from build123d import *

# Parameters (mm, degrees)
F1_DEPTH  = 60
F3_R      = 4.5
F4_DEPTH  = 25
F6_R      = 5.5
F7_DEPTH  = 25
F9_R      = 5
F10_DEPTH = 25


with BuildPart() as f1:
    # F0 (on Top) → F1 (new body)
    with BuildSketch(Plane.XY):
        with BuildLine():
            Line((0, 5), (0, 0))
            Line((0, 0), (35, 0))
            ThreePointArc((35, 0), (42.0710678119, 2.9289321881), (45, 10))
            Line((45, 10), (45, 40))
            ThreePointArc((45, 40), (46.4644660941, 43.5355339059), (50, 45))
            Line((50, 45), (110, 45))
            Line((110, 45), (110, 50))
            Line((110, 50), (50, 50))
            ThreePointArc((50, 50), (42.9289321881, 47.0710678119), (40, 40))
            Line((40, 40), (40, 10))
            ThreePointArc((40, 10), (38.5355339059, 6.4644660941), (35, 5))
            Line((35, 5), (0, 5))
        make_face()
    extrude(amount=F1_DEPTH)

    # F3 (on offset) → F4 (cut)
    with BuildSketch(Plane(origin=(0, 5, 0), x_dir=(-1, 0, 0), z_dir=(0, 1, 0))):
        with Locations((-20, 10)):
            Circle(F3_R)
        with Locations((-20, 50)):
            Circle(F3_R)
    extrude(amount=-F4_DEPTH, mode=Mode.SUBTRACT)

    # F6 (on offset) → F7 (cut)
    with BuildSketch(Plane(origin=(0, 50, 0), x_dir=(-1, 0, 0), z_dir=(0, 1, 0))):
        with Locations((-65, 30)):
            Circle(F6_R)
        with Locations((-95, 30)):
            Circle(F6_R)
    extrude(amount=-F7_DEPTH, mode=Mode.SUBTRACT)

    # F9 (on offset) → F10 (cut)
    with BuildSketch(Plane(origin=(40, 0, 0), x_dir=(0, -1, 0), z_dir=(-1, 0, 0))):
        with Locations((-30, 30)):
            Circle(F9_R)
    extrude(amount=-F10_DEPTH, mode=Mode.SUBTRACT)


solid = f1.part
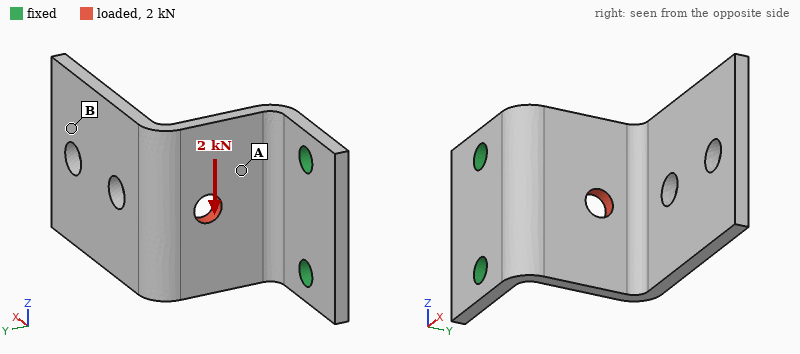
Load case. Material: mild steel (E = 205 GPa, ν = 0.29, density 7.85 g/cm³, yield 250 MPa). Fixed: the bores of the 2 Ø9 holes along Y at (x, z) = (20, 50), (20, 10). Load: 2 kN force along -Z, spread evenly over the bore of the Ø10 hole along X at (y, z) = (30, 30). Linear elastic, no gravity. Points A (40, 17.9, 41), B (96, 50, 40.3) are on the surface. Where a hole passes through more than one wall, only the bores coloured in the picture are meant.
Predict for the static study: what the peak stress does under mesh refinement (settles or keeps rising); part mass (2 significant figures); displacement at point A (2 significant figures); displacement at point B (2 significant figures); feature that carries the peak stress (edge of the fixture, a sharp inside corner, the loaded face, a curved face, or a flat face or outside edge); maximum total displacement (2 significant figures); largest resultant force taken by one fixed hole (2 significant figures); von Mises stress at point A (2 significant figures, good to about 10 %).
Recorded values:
keeps rising
330 g
31 µm
21 µm
edge of the fixture
90 µm
1.9 kN
39 MPa
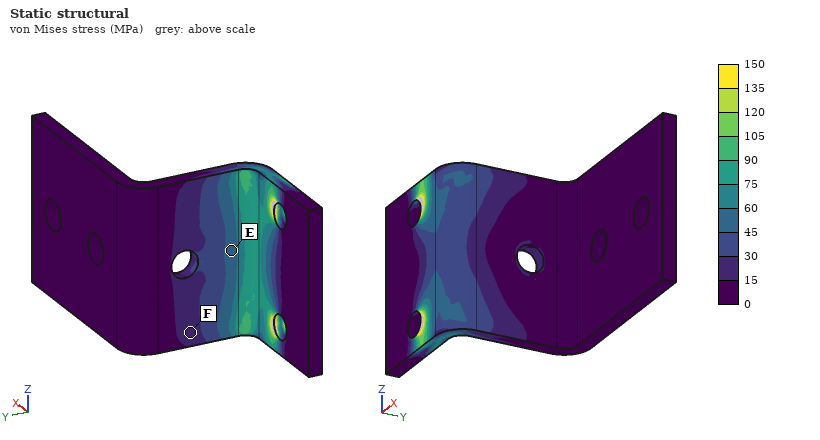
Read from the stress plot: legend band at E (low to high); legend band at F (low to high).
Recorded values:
45 to 60 MPa
15 to 30 MPa
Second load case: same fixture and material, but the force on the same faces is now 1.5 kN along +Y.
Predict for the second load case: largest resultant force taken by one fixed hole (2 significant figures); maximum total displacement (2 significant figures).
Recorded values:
750 N
0.23 mm
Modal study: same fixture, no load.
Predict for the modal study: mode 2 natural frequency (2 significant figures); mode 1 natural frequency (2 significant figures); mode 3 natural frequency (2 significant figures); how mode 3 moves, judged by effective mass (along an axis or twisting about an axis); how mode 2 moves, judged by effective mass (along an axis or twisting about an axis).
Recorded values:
780 Hz
340 Hz
1100 Hz
along X
along Z
